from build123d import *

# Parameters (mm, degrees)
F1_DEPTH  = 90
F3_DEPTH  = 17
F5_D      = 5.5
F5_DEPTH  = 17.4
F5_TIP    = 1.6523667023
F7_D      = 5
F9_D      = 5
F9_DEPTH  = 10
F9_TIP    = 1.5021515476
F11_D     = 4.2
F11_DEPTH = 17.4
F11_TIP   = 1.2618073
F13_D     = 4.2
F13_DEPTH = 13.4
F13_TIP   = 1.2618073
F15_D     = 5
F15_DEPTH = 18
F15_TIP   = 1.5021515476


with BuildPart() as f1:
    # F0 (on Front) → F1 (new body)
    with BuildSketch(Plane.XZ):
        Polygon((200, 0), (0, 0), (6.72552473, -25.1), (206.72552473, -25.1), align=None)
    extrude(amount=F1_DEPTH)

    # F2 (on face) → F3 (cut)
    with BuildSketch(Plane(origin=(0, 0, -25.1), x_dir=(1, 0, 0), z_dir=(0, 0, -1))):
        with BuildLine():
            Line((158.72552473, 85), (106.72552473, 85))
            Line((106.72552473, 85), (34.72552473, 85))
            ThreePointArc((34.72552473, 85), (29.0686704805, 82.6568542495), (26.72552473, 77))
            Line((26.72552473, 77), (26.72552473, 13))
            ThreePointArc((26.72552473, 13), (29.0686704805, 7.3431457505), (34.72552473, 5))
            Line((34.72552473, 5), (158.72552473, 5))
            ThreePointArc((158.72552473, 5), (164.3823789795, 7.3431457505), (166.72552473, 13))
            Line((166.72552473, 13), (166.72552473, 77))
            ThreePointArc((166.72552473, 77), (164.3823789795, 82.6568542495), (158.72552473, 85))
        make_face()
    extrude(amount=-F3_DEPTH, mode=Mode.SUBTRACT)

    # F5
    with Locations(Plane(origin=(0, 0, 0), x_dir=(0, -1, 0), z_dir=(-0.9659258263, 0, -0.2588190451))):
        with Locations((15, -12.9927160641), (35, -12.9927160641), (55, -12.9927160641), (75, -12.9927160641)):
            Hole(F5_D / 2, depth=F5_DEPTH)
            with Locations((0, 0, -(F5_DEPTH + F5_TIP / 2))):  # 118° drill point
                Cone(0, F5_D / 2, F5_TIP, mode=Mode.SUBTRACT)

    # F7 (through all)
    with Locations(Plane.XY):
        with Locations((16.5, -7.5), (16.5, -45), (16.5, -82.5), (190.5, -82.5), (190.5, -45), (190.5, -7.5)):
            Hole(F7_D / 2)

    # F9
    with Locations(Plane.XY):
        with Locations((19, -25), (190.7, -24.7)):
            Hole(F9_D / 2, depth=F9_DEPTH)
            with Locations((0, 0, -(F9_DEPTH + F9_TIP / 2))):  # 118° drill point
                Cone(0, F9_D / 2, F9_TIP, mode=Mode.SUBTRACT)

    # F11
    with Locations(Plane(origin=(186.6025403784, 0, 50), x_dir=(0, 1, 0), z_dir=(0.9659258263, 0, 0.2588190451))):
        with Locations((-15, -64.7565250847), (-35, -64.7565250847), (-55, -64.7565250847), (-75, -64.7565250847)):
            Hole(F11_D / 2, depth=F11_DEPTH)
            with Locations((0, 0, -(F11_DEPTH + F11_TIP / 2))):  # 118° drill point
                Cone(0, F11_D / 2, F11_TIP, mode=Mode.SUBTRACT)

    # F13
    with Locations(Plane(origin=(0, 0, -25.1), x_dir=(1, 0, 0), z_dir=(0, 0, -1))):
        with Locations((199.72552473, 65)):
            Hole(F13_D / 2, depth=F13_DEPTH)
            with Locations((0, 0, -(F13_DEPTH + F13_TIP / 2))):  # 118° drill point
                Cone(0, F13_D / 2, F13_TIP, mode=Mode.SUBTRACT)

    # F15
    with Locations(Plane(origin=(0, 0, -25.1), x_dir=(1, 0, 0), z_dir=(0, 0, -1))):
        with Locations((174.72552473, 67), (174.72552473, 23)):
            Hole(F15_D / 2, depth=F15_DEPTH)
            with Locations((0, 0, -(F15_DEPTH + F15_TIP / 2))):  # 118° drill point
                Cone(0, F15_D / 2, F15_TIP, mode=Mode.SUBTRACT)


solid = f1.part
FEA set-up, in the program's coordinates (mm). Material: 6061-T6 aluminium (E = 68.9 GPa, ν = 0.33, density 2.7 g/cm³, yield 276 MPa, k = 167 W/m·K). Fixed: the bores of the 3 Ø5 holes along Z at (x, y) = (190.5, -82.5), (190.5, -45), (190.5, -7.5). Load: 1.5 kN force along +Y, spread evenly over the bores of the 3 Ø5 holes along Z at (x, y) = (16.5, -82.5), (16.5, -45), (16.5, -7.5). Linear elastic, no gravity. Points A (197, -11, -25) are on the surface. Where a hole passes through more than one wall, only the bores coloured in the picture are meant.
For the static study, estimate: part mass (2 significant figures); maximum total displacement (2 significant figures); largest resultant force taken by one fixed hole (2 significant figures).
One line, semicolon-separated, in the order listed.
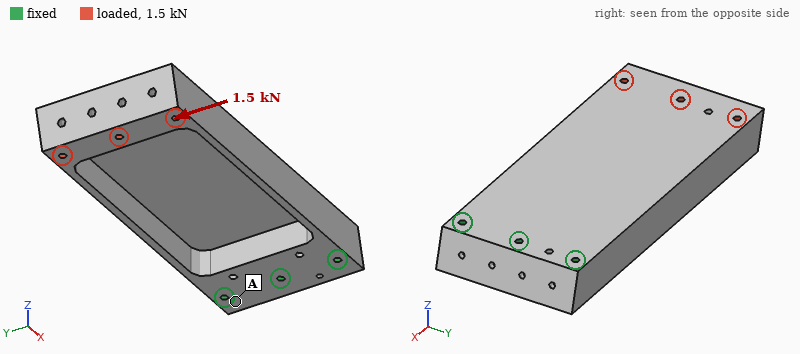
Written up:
690 g; 0.17 mm; 3.5 kN
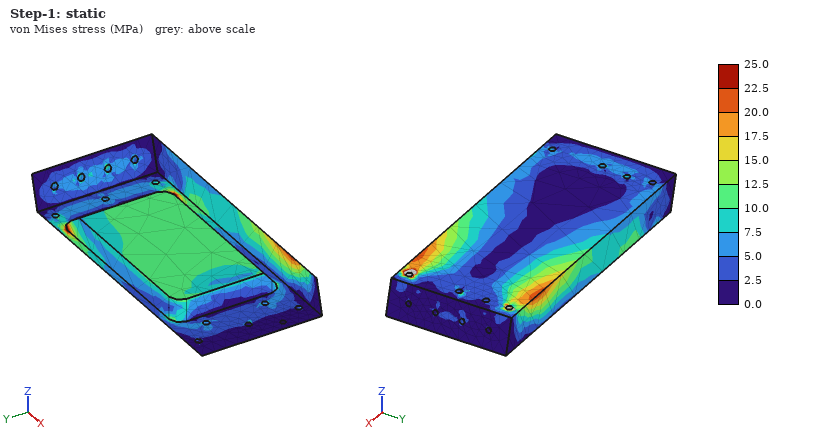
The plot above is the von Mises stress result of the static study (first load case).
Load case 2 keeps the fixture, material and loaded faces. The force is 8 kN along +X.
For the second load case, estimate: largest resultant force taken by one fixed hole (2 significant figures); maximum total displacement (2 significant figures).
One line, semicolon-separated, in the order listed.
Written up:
3.2 kN; 0.36 mm
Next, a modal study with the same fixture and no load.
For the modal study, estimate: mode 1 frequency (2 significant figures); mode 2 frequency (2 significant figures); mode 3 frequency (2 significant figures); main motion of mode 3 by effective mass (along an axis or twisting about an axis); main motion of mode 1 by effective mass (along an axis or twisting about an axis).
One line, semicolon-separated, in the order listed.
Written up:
400 Hz; 920 Hz; 1800 Hz; along Y; along Z
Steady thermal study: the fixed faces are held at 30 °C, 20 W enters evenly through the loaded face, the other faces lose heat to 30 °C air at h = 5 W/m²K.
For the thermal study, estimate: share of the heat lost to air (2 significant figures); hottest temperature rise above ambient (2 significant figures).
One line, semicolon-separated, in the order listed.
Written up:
14 %; 20 K
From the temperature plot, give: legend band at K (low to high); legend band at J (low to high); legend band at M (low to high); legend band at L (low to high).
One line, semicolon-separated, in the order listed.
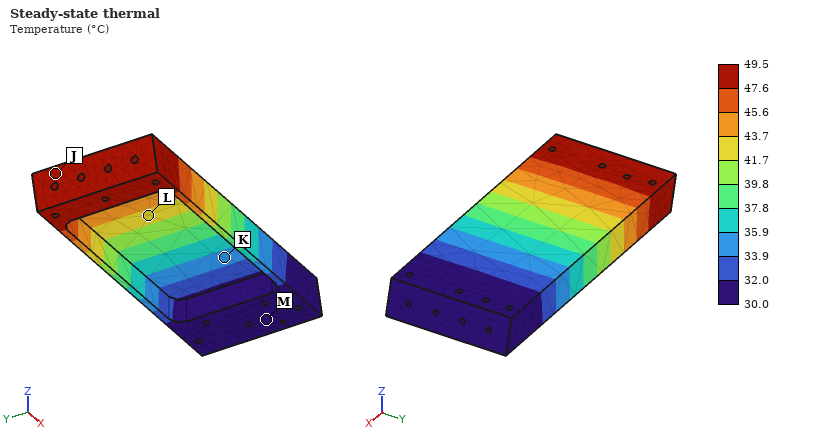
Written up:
33.9 to 35.9 °C; 47.6 to 49.5 °C; 30.0 to 32.0 °C; 41.7 to 43.7 °C
